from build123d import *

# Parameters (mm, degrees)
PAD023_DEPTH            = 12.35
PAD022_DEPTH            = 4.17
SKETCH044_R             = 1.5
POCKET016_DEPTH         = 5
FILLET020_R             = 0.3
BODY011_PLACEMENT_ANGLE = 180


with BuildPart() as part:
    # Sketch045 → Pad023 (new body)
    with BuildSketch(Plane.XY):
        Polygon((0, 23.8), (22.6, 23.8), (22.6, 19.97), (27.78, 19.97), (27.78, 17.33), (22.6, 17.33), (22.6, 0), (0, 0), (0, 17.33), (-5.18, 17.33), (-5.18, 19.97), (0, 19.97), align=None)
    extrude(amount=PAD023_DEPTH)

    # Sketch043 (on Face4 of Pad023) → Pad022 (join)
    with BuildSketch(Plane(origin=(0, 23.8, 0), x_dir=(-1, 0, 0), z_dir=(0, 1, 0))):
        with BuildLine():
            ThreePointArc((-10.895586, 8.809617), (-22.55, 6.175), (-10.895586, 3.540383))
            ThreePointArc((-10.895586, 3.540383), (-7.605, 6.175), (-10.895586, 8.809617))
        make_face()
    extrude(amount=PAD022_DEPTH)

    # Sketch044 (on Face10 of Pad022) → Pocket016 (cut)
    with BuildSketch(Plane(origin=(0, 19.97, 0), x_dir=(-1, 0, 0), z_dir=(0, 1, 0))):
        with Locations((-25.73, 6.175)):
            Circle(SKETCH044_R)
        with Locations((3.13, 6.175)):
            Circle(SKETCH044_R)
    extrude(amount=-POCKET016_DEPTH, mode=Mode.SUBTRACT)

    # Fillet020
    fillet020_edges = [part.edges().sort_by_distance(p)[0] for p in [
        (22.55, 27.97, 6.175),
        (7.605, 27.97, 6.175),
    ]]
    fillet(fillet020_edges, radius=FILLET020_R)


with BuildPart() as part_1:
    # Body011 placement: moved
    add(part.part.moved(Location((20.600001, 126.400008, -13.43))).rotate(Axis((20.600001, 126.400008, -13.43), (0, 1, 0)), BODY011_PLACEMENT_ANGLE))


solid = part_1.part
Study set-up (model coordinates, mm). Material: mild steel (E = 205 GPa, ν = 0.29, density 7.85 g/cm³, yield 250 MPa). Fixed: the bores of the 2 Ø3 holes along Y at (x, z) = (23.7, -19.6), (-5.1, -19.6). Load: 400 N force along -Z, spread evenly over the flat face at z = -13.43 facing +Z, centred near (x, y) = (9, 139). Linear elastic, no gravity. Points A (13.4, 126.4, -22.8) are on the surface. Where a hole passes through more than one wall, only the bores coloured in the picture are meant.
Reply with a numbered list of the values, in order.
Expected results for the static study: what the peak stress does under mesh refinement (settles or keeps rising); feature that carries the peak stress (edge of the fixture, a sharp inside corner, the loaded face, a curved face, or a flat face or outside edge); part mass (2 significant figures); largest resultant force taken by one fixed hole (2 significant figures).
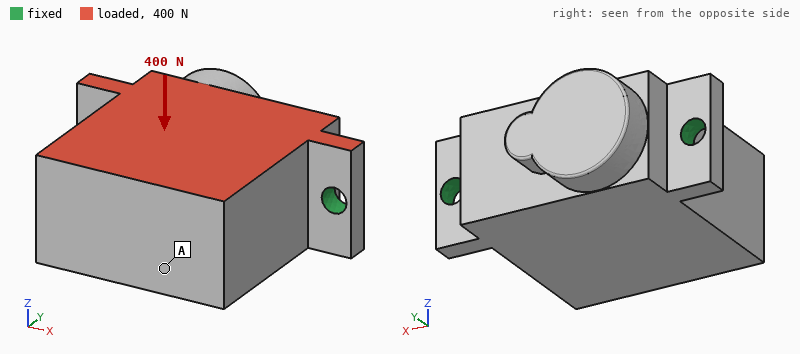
1. keeps rising
2. edge of the fixture
3. 59 g
4. 200 N
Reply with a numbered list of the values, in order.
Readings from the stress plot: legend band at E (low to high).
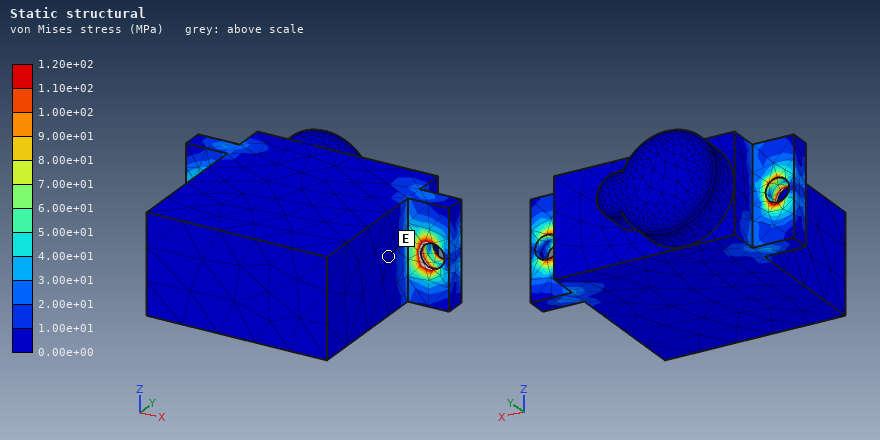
1. 0.00e+00 to 1.00e+01 MPa
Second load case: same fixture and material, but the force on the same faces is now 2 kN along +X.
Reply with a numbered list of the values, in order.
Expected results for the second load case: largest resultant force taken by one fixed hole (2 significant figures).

1. 1.2 kN
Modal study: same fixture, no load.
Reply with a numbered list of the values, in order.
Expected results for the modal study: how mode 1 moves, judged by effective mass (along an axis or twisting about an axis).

1. along Z
